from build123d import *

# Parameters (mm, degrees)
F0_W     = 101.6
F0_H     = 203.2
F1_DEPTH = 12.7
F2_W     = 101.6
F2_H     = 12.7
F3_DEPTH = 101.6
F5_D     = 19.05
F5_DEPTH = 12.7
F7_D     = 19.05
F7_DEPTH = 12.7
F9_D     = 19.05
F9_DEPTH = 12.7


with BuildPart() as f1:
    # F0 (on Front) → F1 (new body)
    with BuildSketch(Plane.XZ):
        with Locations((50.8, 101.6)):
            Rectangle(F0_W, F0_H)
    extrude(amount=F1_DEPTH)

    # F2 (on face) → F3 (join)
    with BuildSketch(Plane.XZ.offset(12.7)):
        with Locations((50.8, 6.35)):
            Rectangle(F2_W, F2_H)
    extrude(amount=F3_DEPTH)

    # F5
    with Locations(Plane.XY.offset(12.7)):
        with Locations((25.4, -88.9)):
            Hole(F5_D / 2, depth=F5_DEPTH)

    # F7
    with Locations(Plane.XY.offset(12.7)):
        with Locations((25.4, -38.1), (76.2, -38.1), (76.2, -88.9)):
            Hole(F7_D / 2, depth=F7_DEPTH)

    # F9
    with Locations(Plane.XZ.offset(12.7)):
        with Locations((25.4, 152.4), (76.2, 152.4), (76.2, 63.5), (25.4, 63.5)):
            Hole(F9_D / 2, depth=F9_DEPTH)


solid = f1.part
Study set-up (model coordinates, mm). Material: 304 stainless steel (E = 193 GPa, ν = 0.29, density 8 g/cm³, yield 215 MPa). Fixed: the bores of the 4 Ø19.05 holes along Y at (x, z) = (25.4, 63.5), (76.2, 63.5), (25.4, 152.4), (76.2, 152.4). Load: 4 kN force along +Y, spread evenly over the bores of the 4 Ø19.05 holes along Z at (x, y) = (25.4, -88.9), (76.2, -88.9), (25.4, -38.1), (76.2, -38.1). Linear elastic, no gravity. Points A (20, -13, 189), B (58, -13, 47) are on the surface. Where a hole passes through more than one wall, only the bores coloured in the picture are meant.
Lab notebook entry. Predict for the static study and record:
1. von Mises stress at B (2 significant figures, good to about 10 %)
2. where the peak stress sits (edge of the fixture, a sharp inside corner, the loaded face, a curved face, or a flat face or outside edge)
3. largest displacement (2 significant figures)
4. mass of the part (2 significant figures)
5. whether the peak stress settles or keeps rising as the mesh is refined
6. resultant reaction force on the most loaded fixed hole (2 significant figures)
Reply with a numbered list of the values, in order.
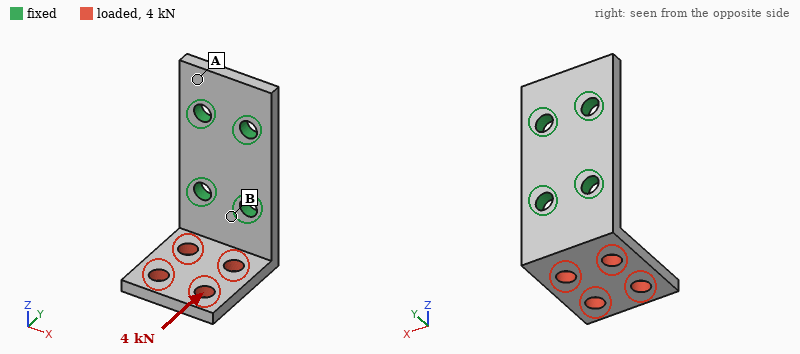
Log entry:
1. 46 MPa
2. edge of the fixture
3. 0.18 mm
4. 2.9 kg
5. keeps rising
6. 2.0 kN
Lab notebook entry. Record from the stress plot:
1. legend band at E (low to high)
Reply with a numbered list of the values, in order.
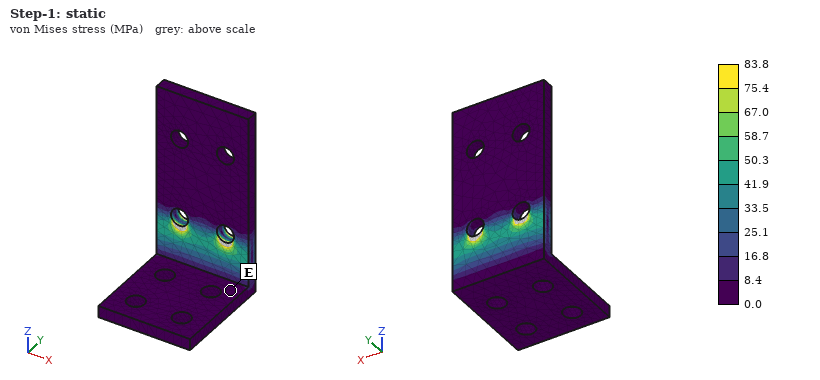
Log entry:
1. 0.0 to 8.4 MPa
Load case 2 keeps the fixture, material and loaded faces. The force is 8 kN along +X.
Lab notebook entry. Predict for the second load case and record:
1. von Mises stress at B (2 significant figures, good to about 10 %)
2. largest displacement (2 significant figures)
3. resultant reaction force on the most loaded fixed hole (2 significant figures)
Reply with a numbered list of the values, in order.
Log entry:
1. 66 MPa
2. 0.28 mm
3. 9.8 kN
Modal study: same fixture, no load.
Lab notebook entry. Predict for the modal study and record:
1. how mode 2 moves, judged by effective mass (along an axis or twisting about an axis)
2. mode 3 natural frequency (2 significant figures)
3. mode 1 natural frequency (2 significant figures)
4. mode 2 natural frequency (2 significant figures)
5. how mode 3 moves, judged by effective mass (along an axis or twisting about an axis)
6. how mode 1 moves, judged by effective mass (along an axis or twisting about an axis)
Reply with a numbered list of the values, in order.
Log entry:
1. along X
2. 1700 Hz
3. 520 Hz
4. 1000 Hz
5. along Y
6. along Z
